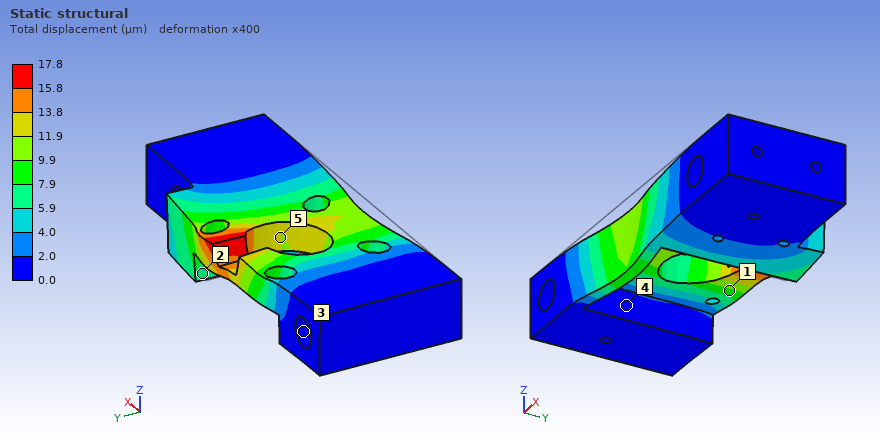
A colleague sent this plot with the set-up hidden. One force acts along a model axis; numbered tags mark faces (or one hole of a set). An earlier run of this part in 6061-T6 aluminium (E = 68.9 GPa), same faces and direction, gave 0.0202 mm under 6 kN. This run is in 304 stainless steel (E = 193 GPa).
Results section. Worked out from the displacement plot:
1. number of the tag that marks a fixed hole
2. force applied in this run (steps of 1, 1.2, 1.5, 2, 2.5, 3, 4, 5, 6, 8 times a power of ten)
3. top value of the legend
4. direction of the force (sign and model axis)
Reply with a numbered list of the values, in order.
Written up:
1. 3
2. 15 kN
3. 17.8 µm
4. +Y
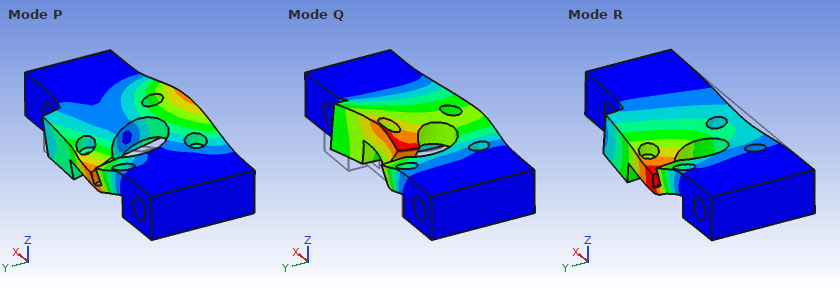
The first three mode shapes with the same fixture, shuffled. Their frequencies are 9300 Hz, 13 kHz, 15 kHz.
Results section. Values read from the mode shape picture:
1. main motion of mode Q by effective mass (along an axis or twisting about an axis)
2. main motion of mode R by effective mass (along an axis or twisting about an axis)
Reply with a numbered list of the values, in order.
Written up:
1. along Y
2. along Z
